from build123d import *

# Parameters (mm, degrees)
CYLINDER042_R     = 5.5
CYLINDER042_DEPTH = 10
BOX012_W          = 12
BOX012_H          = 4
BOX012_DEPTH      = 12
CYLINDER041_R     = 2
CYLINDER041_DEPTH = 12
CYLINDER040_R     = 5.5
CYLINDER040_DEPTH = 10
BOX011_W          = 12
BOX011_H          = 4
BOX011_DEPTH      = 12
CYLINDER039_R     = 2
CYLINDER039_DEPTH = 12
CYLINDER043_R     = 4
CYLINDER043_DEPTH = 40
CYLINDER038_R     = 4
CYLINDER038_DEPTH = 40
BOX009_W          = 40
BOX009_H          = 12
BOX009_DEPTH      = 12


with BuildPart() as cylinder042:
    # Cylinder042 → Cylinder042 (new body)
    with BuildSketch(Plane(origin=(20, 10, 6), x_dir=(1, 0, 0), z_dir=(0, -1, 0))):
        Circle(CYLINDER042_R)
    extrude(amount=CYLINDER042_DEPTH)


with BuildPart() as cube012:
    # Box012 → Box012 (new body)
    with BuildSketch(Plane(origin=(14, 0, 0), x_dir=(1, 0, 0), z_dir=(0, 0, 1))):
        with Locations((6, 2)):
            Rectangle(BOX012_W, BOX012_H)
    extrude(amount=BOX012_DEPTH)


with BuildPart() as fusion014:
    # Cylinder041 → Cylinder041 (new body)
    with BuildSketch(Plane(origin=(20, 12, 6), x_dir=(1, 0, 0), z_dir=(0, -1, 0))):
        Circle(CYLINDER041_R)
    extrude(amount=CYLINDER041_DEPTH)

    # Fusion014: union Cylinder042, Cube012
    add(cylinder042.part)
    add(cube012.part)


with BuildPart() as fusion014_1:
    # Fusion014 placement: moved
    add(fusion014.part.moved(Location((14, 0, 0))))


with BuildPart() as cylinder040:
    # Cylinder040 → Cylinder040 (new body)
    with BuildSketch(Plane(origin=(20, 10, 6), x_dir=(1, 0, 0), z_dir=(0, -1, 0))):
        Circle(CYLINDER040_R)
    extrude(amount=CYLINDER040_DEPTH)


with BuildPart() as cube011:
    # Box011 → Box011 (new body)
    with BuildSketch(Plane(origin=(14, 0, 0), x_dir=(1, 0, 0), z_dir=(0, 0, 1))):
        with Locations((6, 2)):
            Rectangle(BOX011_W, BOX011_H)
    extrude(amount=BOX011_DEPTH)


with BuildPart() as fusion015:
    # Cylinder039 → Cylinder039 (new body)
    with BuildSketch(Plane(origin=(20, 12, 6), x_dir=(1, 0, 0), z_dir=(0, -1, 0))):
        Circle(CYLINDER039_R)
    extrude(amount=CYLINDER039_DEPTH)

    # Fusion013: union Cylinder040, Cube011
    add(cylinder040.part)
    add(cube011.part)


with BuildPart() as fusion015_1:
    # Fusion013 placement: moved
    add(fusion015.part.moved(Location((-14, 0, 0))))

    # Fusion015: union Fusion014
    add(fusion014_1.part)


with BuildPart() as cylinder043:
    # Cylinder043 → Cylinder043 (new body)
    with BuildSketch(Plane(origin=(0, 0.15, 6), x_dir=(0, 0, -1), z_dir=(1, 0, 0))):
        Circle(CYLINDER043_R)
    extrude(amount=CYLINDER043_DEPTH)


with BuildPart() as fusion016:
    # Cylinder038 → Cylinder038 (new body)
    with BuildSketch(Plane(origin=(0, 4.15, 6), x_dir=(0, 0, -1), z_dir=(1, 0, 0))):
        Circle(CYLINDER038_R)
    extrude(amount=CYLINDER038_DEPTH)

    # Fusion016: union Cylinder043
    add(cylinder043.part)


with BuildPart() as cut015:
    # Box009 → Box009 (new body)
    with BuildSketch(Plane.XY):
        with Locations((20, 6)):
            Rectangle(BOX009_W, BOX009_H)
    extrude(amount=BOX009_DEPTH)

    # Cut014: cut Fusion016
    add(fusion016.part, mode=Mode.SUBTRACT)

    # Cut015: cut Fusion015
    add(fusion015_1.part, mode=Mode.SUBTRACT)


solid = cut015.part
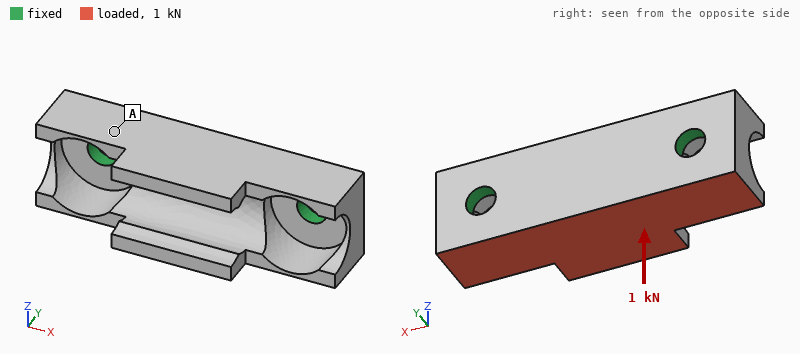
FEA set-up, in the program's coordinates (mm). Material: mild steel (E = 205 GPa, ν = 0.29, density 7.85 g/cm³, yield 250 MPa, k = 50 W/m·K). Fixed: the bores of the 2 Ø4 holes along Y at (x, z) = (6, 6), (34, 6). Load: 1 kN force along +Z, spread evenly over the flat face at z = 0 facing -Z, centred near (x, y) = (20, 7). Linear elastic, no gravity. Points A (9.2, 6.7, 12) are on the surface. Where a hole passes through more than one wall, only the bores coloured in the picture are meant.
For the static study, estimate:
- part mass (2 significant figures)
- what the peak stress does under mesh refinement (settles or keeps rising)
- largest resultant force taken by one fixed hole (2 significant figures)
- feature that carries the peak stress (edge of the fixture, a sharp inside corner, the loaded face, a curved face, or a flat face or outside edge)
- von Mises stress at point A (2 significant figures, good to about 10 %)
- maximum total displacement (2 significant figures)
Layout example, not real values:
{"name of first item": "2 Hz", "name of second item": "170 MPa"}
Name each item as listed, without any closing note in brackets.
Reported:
{"part mass": "19 g", "what the peak stress does under mesh refinement": "keeps rising", "largest resultant force taken by one fixed hole": "500 N", "feature that carries the peak stress": "edge of the fixture", "von Mises stress at point A": "23 MPa", "maximum total displacement": "24 µm"}
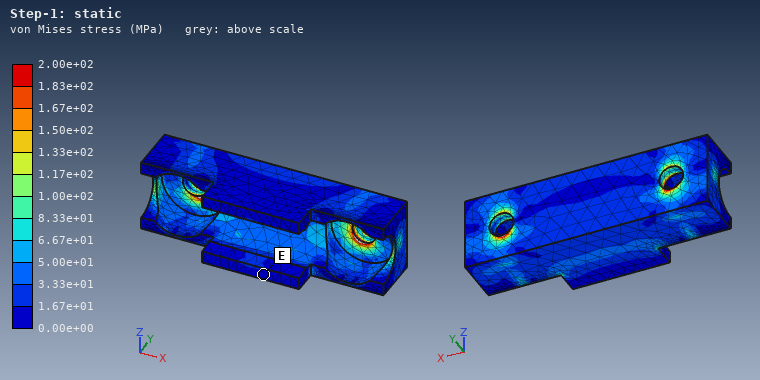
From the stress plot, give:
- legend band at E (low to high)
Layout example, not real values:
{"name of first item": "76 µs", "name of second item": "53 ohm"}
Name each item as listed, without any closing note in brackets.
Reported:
{"legend band at E": "0.00e+00 to 1.67e+01 MPa"}
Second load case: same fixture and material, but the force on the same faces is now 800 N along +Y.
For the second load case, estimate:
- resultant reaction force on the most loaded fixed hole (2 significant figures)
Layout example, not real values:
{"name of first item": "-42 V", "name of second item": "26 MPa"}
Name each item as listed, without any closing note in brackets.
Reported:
{"resultant reaction force on the most loaded fixed hole": "430 N"}
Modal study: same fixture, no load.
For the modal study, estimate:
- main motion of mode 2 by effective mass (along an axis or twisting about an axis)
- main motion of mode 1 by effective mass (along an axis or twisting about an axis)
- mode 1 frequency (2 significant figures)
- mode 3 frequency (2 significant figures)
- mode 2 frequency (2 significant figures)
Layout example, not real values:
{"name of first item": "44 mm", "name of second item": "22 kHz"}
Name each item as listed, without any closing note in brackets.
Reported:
{"main motion of mode 2 by effective mass": "along Y", "main motion of mode 1 by effective mass": "along Z", "mode 1 frequency": "12 kHz", "mode 3 frequency": "26 kHz", "mode 2 frequency": "21 kHz"}
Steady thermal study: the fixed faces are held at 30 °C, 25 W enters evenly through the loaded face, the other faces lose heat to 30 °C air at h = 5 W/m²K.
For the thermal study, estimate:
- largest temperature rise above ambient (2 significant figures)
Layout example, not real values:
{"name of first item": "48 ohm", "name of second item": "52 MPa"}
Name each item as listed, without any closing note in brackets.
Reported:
{"largest temperature rise above ambient": "67 K"}
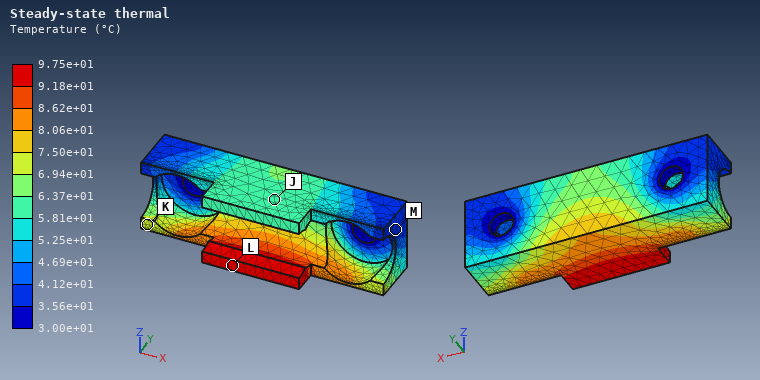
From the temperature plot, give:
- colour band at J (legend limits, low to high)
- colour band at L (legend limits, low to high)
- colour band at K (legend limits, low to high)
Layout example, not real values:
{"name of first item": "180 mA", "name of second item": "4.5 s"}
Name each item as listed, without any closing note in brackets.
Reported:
{"colour band at J": "5.81e+01 to 6.37e+01 °C", "colour band at L": "9.18e+01 to 9.75e+01 °C", "colour band at K": "6.94e+01 to 7.50e+01 °C"}
